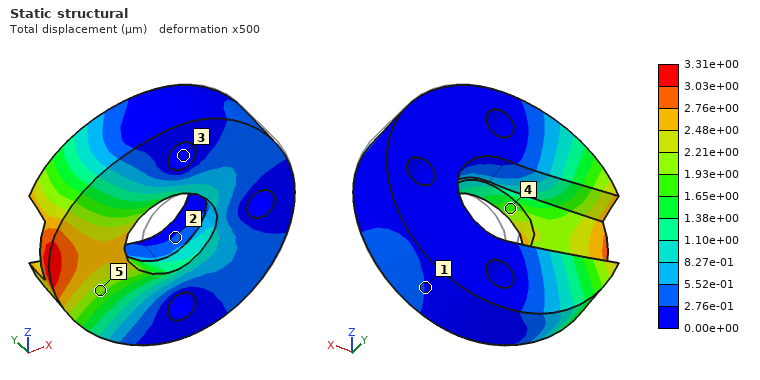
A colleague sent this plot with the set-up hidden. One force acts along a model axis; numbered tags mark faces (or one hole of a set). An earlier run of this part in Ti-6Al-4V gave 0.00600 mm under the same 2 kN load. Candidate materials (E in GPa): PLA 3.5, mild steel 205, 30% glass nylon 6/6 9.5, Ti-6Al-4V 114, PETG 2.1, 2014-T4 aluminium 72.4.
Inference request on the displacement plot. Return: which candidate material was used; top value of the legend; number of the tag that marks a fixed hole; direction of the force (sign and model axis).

mild steel
3.31e+00 µm
3
-X
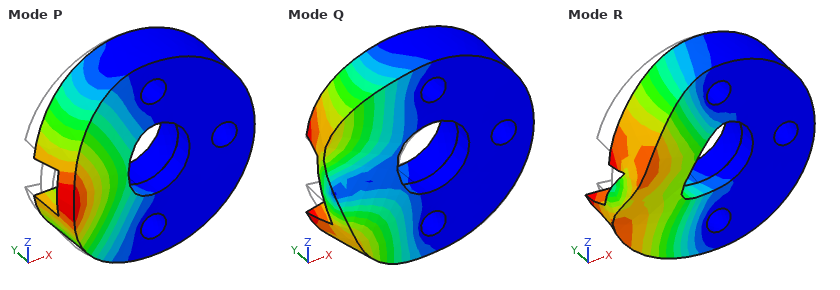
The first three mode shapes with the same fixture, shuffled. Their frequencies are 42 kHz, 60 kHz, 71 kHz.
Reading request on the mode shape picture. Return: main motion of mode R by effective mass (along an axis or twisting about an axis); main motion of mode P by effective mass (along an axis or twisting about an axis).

along Z
along Y
